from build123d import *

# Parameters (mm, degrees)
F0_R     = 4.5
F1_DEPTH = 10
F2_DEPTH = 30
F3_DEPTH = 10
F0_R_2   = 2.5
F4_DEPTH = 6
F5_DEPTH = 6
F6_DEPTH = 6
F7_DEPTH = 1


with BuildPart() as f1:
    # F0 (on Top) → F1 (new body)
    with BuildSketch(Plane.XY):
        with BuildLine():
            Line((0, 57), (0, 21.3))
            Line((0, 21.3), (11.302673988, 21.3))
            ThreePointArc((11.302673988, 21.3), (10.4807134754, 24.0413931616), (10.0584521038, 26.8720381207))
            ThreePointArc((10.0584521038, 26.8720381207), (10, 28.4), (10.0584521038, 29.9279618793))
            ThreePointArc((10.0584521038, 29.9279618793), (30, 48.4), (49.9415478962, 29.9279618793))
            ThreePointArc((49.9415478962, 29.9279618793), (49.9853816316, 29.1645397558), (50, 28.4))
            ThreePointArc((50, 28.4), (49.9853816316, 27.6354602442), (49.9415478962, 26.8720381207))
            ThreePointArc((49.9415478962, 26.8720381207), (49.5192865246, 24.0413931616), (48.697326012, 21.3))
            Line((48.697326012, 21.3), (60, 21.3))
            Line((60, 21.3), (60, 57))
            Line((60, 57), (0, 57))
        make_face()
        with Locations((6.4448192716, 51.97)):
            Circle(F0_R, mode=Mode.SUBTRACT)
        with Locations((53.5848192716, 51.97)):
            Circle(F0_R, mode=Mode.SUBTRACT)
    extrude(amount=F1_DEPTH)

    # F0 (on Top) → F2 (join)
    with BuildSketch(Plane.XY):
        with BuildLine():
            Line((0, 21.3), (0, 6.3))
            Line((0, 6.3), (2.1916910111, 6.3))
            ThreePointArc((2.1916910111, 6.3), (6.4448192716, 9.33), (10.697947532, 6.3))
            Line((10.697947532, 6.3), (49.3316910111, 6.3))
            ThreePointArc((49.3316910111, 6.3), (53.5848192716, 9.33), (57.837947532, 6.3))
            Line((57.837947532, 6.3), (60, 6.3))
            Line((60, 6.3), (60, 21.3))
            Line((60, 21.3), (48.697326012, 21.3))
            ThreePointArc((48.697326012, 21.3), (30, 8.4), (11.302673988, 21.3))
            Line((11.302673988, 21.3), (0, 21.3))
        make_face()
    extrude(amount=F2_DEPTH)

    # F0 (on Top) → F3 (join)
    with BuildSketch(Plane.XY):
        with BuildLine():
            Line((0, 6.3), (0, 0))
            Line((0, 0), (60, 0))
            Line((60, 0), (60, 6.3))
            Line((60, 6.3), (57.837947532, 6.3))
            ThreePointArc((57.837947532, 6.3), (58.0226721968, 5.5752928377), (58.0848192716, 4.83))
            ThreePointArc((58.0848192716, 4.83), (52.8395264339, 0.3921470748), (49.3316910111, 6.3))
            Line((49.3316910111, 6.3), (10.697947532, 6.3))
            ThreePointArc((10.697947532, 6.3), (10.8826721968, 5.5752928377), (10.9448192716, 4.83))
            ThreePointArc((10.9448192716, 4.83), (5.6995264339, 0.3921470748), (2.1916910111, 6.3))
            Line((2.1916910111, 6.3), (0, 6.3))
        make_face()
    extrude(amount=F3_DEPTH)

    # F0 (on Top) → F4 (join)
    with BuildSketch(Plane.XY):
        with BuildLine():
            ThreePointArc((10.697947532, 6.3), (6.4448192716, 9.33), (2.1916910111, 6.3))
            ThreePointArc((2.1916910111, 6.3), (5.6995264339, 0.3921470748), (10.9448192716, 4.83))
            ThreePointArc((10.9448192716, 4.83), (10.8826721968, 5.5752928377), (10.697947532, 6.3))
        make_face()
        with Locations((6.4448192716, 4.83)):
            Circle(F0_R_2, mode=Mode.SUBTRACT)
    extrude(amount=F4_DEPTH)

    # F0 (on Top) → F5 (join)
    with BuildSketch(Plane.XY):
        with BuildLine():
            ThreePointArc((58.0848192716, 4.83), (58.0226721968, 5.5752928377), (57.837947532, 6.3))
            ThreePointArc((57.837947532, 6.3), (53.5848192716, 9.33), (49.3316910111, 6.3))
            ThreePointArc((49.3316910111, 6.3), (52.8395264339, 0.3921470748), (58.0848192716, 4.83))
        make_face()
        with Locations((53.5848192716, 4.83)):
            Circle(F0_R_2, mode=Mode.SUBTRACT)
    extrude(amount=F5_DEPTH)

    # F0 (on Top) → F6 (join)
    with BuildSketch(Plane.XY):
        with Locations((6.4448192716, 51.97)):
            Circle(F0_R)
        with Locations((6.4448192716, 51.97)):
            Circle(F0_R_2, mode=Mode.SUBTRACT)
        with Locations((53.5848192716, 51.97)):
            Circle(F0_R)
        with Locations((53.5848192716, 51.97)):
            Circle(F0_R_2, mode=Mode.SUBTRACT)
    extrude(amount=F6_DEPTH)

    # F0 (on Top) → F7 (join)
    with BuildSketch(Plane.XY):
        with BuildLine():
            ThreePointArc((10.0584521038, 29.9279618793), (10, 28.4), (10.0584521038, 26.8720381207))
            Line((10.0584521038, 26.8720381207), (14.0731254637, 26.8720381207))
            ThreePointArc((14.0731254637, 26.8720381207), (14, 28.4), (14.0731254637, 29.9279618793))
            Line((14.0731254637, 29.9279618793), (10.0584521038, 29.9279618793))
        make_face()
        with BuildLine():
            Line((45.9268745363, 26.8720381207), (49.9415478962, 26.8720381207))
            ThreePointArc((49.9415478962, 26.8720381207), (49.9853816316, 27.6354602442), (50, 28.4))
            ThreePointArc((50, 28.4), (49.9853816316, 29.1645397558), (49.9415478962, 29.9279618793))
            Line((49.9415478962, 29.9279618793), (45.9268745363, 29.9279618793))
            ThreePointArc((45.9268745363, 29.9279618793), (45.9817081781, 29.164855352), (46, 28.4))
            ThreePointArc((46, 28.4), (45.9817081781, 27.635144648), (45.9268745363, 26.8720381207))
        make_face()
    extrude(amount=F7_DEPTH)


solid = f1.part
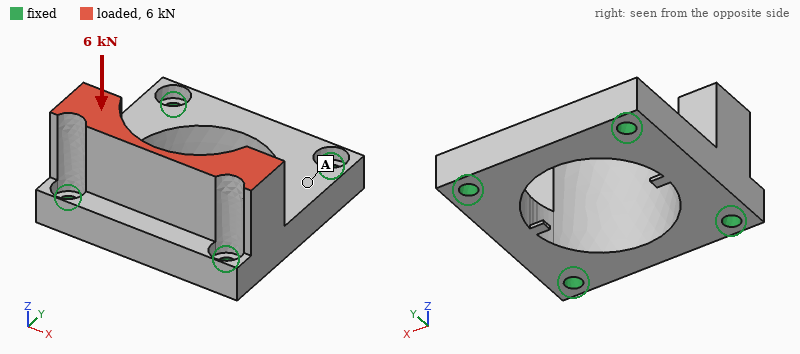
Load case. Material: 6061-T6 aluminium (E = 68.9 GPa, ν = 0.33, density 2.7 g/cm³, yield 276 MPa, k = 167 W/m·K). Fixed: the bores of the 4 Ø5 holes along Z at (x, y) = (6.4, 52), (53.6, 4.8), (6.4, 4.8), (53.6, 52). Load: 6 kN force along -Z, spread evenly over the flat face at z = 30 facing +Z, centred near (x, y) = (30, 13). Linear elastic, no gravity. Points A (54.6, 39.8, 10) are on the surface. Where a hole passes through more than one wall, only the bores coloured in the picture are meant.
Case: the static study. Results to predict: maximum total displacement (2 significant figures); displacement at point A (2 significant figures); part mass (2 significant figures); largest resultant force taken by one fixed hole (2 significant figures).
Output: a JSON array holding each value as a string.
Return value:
["29 µm", "7.9 µm", "82 g", "2.7 kN"]
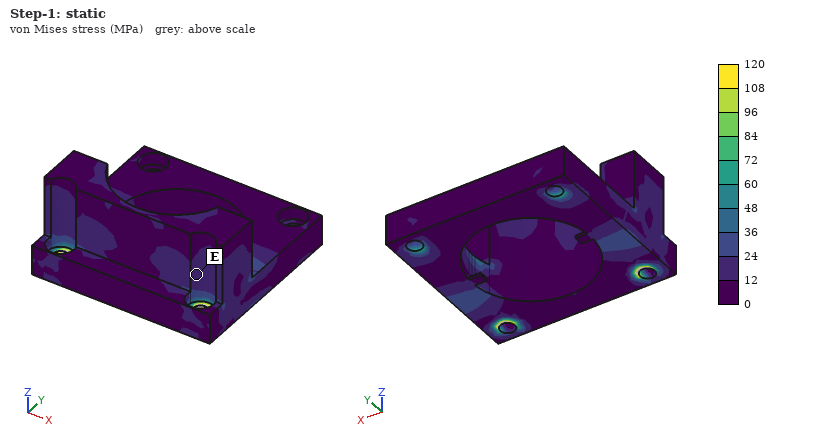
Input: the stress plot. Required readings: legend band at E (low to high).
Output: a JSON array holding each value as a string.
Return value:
["12 to 24 MPa"]
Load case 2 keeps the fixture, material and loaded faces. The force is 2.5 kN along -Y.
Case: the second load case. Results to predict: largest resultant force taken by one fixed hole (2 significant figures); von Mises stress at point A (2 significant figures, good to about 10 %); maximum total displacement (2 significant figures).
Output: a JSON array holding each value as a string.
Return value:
["1.1 kN", "12 MPa", "82 µm"]
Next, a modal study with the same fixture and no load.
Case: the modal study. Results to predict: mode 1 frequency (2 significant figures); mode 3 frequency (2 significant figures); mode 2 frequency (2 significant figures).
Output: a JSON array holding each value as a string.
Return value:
["8100 Hz", "12 kHz", "9400 Hz"]
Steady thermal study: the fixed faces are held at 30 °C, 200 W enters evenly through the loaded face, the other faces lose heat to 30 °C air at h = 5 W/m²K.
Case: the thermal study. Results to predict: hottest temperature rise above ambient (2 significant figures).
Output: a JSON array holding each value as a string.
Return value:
["80 K"]
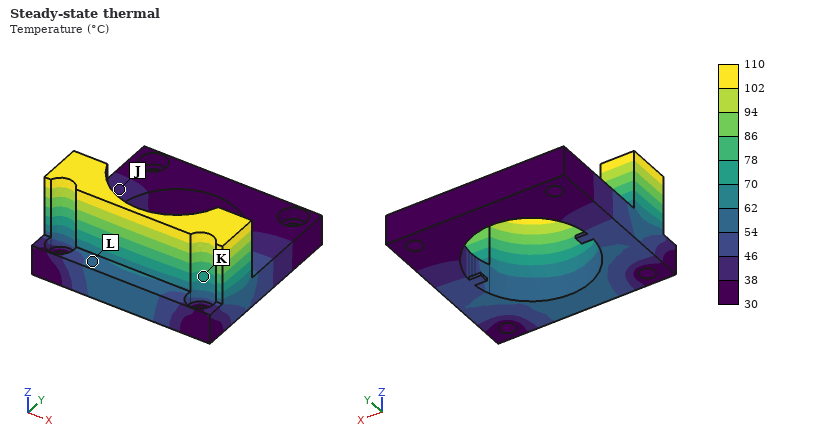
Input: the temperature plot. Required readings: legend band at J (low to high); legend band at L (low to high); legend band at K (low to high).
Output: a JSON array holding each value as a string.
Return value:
["38 to 46 °C", "54 to 62 °C", "70 to 78 °C"]
